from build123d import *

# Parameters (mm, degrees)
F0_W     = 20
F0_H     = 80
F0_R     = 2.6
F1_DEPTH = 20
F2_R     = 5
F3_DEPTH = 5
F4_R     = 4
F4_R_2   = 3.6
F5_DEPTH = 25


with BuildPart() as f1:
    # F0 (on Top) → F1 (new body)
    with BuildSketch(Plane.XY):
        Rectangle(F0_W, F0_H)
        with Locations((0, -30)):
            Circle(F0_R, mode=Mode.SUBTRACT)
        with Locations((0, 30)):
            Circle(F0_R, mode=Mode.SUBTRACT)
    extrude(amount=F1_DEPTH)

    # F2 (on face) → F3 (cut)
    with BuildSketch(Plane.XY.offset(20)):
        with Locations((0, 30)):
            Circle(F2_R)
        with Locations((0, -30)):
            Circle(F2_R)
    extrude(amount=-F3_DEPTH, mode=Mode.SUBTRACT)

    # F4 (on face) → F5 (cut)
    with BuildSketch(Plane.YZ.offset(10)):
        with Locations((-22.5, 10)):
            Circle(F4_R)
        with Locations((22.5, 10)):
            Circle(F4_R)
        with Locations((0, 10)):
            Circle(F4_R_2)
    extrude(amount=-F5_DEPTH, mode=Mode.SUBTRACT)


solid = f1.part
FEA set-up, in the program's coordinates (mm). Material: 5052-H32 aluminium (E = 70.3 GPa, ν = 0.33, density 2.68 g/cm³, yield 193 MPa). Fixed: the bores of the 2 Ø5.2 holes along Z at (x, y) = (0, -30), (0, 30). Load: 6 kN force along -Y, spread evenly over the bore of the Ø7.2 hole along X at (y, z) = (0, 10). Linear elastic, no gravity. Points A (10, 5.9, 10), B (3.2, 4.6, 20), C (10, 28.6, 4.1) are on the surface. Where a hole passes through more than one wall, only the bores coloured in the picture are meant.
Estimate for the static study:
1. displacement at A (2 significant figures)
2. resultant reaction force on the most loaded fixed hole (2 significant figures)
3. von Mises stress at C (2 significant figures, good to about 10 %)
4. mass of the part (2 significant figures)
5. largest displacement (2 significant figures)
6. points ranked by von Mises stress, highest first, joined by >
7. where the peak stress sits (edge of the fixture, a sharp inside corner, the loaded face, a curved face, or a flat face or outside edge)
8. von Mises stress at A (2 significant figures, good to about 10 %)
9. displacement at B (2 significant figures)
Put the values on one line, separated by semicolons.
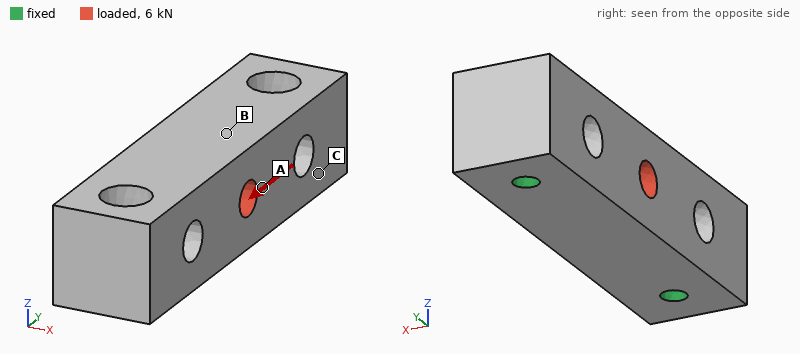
5.1 µm; 3.0 kN; 7.3 MPa; 74 g; 5.8 µm; A > C > B; a curved face; 13 MPa; 4.3 µm
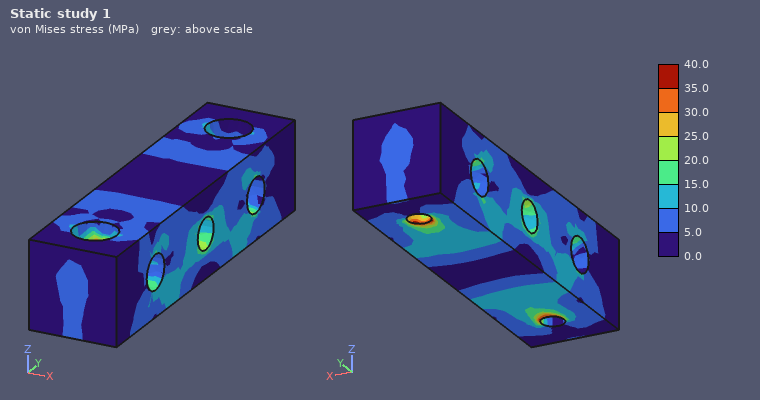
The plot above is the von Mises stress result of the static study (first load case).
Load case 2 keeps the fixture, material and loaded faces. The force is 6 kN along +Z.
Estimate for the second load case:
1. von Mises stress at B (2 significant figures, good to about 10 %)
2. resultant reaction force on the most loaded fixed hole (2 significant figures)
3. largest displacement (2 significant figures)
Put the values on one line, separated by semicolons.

39 MPa; 3.2 kN; 29 µm
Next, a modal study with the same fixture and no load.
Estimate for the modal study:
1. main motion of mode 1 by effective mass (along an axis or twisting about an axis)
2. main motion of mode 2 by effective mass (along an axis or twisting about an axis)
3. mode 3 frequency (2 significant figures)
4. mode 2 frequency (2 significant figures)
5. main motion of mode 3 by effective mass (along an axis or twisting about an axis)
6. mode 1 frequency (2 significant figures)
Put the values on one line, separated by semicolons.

along X; along Z; 19 kHz; 14 kHz; twisting about Y; 13 kHz
